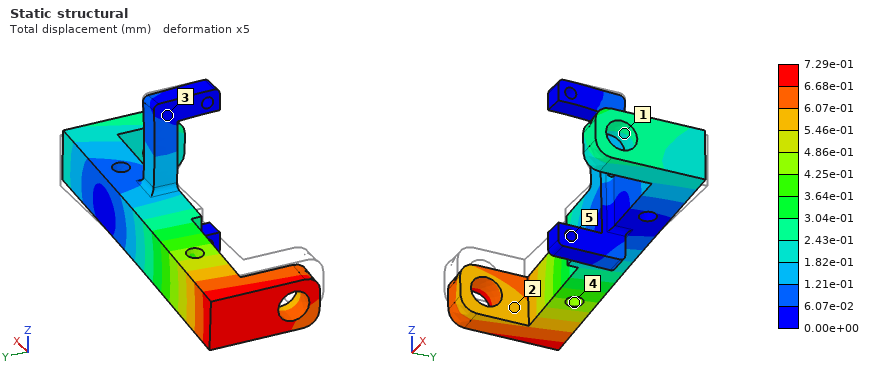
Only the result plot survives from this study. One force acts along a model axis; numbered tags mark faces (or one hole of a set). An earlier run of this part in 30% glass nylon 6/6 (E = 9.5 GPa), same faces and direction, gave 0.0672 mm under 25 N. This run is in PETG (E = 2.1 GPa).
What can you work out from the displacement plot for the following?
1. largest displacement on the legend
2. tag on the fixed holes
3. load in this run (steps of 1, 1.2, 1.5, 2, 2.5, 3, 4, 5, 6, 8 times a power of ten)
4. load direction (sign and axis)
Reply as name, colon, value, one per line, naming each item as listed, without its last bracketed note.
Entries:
largest displacement on the legend: 7.29e-01 mm
tag on the fixed holes: 5
load in this run: 60 N
load direction: -Z
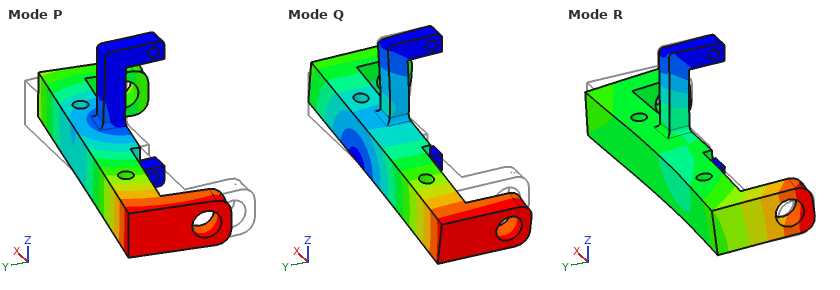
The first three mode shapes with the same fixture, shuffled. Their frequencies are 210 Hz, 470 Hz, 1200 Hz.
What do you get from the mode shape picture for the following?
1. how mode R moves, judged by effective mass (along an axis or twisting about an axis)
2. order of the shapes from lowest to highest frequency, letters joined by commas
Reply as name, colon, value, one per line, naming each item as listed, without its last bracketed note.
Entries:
how mode R moves, judged by effective mass: along X
order of the shapes from lowest to highest frequency, letters joined by commas: P, Q, R
